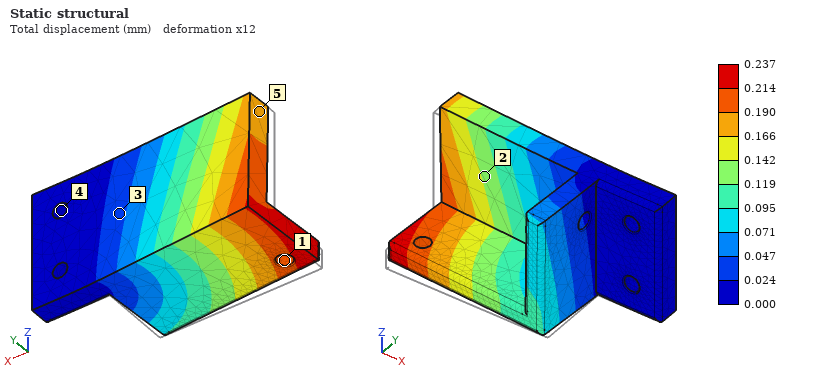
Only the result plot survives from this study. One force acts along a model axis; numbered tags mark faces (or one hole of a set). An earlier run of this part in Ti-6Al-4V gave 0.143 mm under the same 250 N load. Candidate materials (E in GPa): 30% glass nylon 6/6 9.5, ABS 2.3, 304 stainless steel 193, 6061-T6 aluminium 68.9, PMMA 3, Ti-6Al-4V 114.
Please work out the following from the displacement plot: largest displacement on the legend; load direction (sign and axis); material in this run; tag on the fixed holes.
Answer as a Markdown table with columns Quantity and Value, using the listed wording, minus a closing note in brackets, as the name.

| Quantity | Value |
|---|---|
| largest displacement on the legend | 0.237 mm |
| load direction | +Y |
| material in this run | 6061-T6 aluminium |
| tag on the fixed holes | 4 |
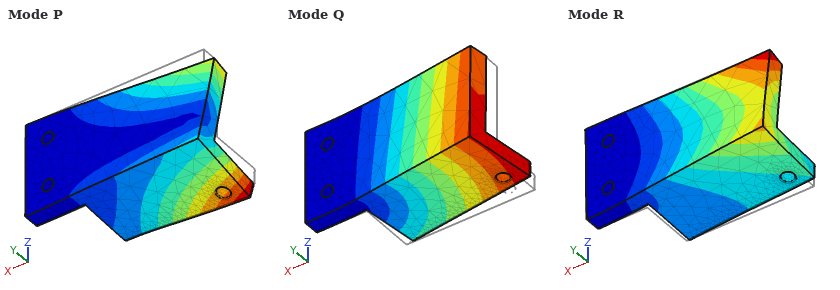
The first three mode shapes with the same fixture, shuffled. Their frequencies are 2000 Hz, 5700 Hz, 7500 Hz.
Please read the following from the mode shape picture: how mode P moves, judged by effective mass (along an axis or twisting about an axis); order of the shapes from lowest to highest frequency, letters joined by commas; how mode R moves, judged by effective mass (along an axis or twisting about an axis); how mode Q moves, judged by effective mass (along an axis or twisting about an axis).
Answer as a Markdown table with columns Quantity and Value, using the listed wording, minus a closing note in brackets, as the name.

| Quantity | Value |
|---|---|
| how mode P moves, judged by effective mass | along Z |
| order of the shapes from lowest to highest frequency, letters joined by commas | Q, P, R |
| how mode R moves, judged by effective mass | along Z |
| how mode Q moves, judged by effective mass | along Y |
